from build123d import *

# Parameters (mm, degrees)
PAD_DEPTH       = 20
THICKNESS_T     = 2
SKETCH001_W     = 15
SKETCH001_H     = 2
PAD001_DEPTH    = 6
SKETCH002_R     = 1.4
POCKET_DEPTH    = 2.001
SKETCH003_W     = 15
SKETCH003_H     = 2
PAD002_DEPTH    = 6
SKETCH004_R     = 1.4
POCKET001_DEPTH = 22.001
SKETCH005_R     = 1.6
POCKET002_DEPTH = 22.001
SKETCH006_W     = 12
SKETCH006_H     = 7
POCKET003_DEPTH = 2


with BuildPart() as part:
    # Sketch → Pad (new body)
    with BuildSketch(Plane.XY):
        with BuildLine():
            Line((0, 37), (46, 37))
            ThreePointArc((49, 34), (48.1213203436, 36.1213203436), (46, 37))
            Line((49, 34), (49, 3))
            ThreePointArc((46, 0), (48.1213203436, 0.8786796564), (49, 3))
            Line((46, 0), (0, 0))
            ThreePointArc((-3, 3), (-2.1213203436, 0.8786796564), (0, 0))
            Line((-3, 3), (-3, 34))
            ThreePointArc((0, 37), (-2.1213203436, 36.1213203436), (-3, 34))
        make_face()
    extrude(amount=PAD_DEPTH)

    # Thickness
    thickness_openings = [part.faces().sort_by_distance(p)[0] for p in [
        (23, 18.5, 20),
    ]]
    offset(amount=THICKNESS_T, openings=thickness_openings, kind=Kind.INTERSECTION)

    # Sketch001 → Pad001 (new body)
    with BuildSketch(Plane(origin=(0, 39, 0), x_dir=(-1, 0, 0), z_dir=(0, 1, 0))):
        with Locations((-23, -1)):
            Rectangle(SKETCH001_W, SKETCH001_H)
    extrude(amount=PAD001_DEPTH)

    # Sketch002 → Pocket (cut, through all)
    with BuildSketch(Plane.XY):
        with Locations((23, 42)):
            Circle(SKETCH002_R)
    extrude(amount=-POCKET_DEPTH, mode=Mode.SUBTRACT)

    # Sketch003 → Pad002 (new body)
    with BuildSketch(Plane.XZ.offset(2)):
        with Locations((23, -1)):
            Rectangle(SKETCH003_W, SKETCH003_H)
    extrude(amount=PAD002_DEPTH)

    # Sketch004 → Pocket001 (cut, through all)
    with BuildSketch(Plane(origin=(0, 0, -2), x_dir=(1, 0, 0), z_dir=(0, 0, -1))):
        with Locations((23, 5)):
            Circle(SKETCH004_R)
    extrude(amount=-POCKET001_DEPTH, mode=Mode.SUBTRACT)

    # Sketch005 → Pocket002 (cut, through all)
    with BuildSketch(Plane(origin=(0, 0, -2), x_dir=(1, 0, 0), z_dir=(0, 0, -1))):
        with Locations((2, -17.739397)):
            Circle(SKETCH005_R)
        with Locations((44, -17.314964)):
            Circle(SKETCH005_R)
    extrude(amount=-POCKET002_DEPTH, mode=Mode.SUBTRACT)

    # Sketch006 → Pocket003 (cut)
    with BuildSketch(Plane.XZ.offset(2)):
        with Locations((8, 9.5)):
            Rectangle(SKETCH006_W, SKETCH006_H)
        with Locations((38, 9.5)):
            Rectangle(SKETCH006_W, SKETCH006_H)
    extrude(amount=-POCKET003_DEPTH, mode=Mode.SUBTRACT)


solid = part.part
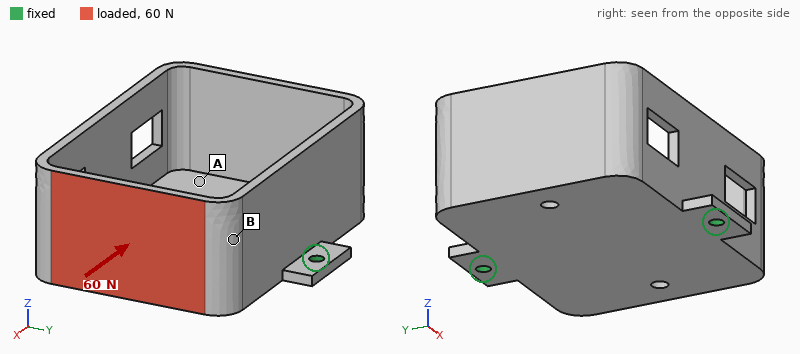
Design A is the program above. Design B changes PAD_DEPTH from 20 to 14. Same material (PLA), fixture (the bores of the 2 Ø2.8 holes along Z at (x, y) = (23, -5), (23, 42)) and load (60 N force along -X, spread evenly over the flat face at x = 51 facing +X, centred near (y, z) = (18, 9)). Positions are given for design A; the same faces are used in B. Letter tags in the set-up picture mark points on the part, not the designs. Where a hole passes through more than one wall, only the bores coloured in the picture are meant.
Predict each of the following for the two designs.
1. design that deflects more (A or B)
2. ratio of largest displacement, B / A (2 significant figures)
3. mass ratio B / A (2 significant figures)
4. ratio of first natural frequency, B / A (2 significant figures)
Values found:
A
0.70
0.82
1.2
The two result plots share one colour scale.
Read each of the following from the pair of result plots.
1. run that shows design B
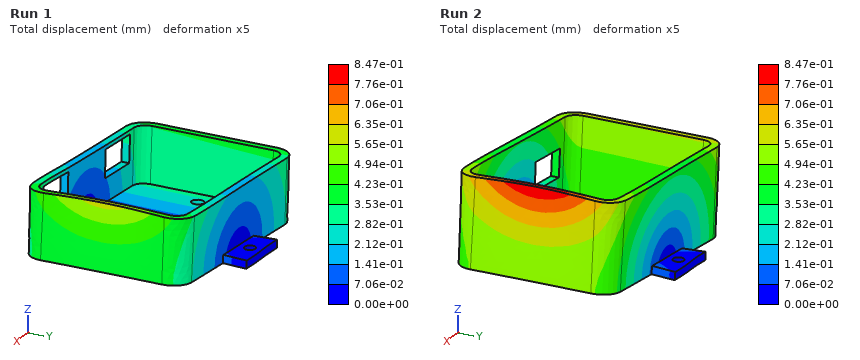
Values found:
Run 1
